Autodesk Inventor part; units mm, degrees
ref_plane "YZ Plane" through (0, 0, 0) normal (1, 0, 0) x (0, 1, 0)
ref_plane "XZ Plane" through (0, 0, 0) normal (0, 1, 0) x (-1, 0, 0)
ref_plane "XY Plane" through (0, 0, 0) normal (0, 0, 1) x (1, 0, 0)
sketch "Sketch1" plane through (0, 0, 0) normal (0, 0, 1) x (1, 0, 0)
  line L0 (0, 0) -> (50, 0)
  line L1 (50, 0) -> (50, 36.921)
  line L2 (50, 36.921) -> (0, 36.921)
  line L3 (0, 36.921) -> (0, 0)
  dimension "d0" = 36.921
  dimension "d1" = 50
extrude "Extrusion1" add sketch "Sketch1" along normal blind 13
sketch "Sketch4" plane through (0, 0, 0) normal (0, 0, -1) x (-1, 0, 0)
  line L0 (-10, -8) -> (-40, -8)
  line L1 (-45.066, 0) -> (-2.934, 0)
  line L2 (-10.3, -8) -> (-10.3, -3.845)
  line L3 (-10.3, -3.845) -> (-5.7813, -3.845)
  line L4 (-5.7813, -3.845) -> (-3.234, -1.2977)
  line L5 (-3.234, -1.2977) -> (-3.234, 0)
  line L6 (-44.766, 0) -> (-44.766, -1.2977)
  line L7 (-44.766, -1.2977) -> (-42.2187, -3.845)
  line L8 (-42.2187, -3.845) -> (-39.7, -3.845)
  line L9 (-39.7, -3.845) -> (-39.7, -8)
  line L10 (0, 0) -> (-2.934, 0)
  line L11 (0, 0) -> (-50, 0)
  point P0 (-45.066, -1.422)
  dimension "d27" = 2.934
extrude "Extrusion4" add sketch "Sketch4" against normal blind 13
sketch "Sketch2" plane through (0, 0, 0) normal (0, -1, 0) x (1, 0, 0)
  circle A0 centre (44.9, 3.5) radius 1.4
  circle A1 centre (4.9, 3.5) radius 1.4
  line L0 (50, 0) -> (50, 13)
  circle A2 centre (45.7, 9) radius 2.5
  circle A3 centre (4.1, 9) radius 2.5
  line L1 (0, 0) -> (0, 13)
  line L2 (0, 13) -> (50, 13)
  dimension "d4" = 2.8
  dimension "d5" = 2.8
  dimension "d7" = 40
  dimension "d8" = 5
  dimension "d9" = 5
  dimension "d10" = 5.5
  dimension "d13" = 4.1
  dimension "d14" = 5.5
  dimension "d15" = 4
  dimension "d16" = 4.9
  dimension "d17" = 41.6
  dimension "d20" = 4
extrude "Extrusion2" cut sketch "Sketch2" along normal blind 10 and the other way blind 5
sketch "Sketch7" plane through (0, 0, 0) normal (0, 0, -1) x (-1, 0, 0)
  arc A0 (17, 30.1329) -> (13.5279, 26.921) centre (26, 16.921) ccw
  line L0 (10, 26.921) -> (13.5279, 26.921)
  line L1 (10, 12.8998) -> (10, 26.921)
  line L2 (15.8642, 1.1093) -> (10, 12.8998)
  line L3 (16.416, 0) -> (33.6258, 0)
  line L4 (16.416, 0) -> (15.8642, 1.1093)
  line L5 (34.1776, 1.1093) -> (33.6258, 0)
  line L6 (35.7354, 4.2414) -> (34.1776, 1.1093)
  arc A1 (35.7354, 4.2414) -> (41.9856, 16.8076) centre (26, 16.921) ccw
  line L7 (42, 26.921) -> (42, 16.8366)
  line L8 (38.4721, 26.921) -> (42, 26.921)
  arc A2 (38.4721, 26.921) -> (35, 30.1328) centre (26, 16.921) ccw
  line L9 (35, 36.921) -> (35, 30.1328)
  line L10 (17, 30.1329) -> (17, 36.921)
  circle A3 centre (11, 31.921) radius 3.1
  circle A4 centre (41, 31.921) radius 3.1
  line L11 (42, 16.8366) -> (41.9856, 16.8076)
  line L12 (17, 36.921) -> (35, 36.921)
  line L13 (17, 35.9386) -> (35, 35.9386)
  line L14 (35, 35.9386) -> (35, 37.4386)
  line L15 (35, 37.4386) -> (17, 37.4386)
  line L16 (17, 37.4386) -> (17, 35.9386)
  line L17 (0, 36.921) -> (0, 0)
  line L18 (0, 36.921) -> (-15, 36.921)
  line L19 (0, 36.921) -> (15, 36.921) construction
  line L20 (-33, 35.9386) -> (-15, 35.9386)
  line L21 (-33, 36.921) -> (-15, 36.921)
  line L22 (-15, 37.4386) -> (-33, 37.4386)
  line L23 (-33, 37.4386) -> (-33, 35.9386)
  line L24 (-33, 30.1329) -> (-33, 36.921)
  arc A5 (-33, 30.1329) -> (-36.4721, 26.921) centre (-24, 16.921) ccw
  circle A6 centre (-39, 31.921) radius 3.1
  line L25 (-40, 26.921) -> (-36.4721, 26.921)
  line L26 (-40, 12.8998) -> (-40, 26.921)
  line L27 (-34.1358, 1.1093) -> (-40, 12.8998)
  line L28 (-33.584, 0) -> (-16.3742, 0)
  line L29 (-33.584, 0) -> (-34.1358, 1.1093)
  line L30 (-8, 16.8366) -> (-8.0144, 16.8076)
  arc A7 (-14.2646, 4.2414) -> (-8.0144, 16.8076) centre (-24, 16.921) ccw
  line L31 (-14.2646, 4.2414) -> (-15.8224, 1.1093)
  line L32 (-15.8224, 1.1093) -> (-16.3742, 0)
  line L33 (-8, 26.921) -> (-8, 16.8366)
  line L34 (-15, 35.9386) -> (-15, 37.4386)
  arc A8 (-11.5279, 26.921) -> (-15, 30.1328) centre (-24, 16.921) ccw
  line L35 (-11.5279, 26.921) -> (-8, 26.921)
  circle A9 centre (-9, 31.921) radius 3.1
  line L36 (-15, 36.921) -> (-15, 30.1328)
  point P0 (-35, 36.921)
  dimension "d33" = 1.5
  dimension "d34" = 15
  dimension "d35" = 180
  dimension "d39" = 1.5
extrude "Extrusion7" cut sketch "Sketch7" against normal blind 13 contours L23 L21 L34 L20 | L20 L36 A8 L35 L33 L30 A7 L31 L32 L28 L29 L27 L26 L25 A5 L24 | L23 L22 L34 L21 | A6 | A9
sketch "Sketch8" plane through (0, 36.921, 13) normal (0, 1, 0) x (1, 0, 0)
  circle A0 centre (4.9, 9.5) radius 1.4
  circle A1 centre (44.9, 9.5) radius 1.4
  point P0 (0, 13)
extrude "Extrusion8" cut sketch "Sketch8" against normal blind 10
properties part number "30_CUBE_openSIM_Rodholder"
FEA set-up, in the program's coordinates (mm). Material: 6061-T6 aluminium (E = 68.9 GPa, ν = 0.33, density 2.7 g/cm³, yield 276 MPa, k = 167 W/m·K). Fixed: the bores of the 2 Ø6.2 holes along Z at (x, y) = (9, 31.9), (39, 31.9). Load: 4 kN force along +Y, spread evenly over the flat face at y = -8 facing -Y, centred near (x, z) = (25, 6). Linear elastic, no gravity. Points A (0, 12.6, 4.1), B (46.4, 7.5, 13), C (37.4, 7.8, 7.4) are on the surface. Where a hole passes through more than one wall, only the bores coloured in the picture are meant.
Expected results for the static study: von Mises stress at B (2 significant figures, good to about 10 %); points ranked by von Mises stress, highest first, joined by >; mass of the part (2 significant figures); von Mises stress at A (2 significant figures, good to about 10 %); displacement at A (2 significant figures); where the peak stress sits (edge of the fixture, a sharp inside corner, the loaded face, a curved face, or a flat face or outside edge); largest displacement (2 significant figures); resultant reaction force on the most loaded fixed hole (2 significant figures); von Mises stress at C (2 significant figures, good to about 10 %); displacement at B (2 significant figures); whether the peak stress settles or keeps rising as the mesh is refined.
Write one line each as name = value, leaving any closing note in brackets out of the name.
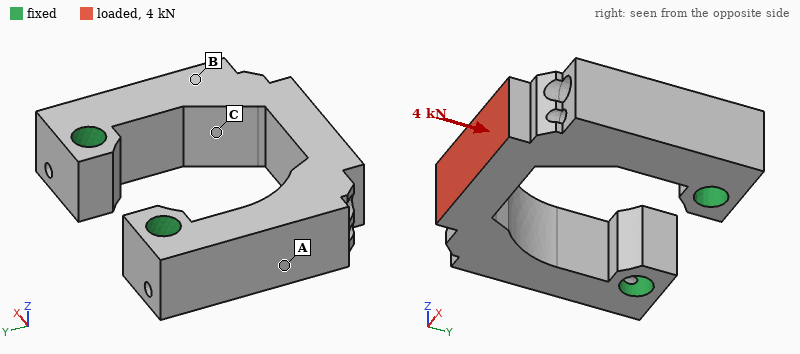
von Mises stress at B = 10 MPa
points ranked by von Mises stress, highest first, joined by > = C > A > B
mass of the part = 38 g
von Mises stress at A = 26 MPa
displacement at A = 17 µm
where the peak stress sits = edge of the fixture
largest displacement = 36 µm
resultant reaction force on the most loaded fixed hole = 2.2 kN
von Mises stress at C = 49 MPa
displacement at B = 15 µm
whether the peak stress settles or keeps rising as the mesh is refined = keeps rising
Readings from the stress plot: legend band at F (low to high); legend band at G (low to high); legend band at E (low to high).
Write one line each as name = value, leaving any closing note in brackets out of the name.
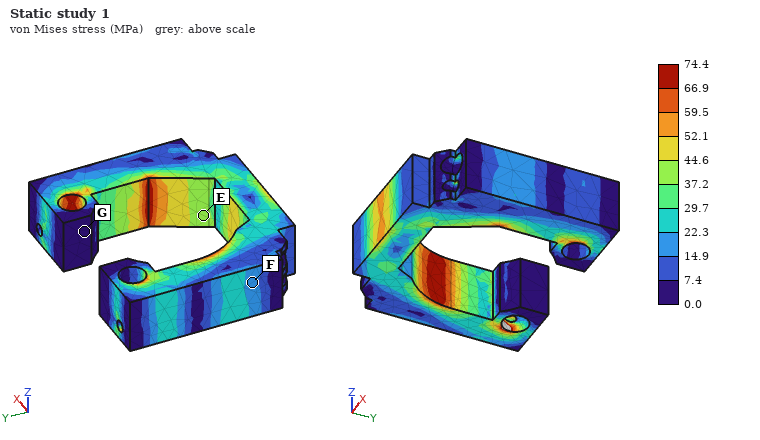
legend band at F = 14.9 to 22.3 MPa
legend band at G = 0.0 to 7.4 MPa
legend band at E = 37.2 to 44.6 MPa
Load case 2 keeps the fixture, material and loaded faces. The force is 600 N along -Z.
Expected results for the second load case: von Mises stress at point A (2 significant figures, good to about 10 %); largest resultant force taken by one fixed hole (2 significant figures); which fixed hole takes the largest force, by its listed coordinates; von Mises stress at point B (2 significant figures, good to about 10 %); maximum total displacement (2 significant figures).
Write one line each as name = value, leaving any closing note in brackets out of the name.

von Mises stress at point A = 7.6 MPa
largest resultant force taken by one fixed hole = 320 N
which fixed hole takes the largest force, by its listed coordinates = (39, 31.9)
von Mises stress at point B = 13 MPa
maximum total displacement = 75 µm
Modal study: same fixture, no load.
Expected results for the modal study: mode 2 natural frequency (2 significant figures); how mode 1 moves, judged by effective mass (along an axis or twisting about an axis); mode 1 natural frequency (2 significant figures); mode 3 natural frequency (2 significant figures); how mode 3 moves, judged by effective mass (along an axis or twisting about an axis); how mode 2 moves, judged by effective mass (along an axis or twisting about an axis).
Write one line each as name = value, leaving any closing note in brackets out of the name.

mode 2 natural frequency = 5800 Hz
how mode 1 moves, judged by effective mass = along Z
mode 1 natural frequency = 4600 Hz
mode 3 natural frequency = 9600 Hz
how mode 3 moves, judged by effective mass = twisting about Y
how mode 2 moves, judged by effective mass = along X
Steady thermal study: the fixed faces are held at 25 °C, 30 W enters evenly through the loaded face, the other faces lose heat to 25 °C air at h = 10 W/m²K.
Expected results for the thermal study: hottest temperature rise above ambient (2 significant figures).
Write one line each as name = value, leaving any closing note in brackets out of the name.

hottest temperature rise above ambient = 32 K
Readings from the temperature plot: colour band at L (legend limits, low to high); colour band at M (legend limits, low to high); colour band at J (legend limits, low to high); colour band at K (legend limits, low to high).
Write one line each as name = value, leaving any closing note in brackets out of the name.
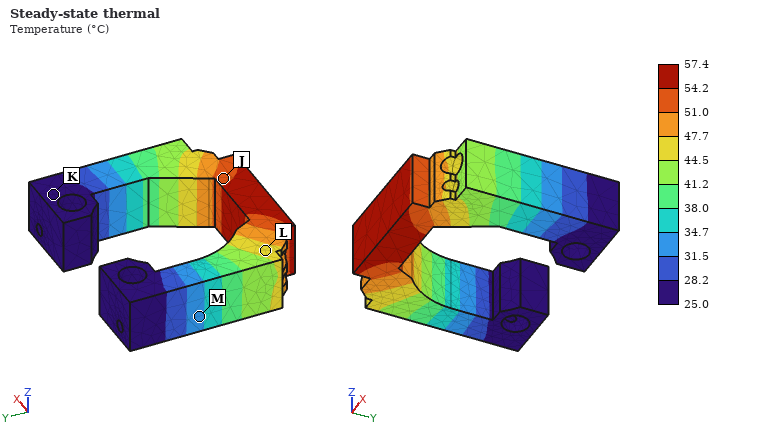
colour band at L = 44.5 to 47.7 °C
colour band at M = 31.5 to 34.7 °C
colour band at J = 51.0 to 54.2 °C
colour band at K = 25.0 to 28.2 °C
